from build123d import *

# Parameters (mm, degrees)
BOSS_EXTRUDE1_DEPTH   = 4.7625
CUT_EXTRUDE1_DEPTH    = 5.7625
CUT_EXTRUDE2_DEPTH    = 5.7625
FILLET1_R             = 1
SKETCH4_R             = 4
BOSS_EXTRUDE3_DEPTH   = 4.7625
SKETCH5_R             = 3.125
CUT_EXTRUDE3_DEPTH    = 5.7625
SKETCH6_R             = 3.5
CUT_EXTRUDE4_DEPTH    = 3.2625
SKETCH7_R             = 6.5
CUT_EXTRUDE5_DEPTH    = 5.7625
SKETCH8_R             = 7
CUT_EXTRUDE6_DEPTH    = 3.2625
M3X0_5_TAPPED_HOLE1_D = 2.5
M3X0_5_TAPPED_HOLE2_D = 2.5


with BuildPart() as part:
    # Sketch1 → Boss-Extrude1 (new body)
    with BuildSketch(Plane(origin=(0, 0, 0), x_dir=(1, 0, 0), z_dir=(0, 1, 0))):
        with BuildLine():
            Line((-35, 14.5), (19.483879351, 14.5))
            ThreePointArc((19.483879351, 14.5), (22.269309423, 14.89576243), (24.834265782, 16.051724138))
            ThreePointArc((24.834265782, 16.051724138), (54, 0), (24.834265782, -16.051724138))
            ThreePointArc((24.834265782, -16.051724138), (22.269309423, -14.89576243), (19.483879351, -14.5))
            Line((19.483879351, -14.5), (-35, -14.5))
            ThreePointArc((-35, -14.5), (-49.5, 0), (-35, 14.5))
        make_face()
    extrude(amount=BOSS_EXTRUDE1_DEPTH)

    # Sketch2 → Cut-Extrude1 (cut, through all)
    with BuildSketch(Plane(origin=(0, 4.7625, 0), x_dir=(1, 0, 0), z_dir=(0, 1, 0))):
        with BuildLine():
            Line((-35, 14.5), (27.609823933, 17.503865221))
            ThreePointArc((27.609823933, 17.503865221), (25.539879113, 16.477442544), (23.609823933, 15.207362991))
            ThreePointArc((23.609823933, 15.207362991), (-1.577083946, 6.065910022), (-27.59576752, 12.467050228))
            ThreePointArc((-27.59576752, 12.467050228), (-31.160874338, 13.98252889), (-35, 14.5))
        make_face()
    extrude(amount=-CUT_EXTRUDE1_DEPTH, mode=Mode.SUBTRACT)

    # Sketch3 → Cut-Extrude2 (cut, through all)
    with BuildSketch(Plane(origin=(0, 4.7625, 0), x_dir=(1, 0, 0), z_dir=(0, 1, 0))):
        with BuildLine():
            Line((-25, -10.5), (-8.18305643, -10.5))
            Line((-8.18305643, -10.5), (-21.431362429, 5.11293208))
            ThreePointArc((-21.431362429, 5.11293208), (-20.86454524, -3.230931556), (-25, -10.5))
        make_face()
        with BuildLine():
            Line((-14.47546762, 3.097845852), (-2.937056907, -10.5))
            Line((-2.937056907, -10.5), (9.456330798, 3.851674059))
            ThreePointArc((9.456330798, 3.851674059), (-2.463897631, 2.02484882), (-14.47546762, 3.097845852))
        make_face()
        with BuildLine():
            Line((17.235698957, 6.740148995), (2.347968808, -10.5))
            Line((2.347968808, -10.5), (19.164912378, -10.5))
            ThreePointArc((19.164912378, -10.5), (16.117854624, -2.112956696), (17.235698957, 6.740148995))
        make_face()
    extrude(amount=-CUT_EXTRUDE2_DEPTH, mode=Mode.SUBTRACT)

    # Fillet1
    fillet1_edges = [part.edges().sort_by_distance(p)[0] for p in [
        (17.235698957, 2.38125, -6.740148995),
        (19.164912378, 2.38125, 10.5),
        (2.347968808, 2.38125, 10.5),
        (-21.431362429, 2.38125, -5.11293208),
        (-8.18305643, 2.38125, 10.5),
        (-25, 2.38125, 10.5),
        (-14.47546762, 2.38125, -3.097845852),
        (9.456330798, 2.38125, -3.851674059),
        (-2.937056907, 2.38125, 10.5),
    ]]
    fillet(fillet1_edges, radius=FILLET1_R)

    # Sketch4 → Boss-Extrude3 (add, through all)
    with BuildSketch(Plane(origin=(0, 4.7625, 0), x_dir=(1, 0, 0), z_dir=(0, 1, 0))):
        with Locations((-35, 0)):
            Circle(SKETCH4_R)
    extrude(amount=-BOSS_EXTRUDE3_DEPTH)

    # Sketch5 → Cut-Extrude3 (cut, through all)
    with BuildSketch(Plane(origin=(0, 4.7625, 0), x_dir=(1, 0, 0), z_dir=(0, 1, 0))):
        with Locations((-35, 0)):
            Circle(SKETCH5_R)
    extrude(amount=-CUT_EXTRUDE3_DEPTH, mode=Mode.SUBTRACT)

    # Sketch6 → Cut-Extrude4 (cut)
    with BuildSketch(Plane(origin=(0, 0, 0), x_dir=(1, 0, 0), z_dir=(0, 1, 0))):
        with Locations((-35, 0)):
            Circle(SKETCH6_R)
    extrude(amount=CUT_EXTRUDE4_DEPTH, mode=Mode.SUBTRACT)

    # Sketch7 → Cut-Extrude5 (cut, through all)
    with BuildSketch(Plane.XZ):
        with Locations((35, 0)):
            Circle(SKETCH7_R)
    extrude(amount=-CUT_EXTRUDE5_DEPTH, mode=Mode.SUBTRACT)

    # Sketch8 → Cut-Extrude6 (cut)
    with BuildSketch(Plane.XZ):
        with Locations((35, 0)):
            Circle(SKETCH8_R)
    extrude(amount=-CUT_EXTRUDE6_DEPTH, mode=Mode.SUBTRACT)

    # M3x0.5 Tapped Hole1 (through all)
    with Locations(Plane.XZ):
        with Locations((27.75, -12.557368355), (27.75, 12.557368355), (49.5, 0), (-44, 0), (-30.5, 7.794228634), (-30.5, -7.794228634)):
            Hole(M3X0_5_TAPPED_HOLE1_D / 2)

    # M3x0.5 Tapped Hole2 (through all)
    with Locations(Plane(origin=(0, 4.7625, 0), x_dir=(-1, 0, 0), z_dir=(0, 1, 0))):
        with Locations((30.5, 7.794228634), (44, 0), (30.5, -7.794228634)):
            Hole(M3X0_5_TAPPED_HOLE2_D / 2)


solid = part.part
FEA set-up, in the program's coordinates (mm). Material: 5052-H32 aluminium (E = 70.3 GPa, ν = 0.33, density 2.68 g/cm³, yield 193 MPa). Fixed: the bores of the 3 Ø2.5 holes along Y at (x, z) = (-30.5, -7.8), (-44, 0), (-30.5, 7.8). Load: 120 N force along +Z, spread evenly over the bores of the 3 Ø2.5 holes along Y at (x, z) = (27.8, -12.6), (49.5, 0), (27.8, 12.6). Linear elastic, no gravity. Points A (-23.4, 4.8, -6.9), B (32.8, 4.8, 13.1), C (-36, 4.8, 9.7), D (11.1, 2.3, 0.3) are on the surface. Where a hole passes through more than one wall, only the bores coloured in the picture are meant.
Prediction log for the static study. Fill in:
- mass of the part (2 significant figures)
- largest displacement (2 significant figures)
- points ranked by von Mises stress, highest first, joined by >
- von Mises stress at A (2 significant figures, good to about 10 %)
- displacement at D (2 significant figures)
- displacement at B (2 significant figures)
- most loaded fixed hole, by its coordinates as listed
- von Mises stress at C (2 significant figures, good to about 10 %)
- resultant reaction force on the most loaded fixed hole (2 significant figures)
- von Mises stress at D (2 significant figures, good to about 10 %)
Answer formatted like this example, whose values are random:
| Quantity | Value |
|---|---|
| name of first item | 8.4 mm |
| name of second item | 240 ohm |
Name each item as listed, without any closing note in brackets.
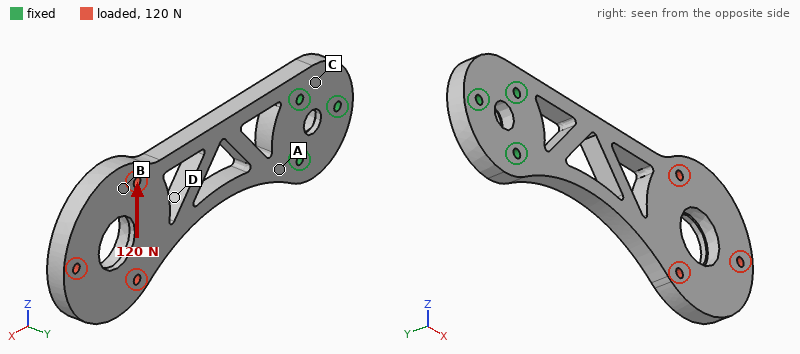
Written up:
| Quantity | Value |
|---|---|
| mass of the part | 27 g |
| largest displacement | 84 µm |
| points ranked by von Mises stress, highest first, joined by > | D > A > C > B |
| von Mises stress at A | 12 MPa |
| displacement at D | 29 µm |
| displacement at B | 59 µm |
| most loaded fixed hole, by its coordinates as listed | (-30.5, -7.8) |
| von Mises stress at C | 4.9 MPa |
| resultant reaction force on the most loaded fixed hole | 430 N |
| von Mises stress at D | 21 MPa |
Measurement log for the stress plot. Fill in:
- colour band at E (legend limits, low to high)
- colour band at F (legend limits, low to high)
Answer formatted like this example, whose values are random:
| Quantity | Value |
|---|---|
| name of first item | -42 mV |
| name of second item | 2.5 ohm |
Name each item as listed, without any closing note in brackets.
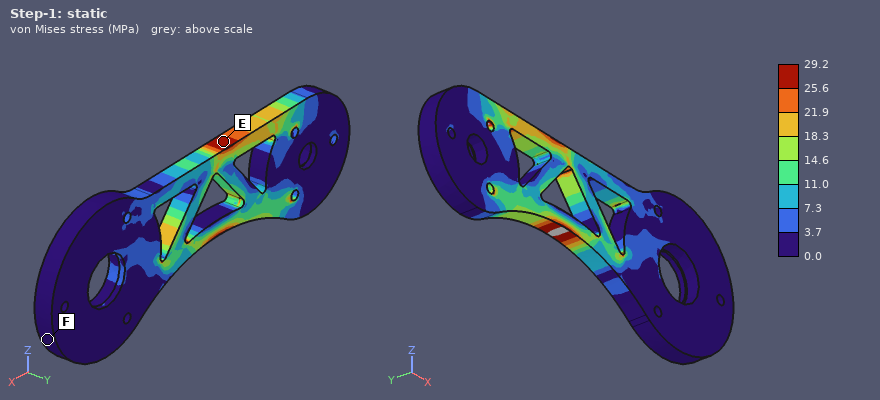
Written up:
| Quantity | Value |
|---|---|
| colour band at E | 25.6 to 29.2 MPa |
| colour band at F | 0.0 to 3.7 MPa |
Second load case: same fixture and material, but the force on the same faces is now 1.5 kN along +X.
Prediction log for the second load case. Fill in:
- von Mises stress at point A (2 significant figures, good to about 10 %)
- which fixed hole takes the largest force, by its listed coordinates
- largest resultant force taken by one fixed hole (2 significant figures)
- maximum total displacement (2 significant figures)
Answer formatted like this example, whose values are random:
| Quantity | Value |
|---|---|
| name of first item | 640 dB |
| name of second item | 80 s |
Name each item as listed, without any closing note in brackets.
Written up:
| Quantity | Value |
|---|---|
| von Mises stress at point A | 25 MPa |
| which fixed hole takes the largest force, by its listed coordinates | (-30.5, -7.8) |
| largest resultant force taken by one fixed hole | 780 N |
| maximum total displacement | 82 µm |
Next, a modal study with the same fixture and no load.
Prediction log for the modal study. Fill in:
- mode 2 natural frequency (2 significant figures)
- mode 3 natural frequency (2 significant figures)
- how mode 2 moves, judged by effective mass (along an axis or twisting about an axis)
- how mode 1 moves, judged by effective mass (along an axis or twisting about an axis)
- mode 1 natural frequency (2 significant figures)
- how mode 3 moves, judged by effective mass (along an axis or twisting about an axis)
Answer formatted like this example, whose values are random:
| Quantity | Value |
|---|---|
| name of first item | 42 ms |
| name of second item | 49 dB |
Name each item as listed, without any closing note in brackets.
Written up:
| Quantity | Value |
|---|---|
| mode 2 natural frequency | 1700 Hz |
| mode 3 natural frequency | 1900 Hz |
| how mode 2 moves, judged by effective mass | twisting about X |
| how mode 1 moves, judged by effective mass | along Y |
| mode 1 natural frequency | 380 Hz |
| how mode 3 moves, judged by effective mass | along Z |
